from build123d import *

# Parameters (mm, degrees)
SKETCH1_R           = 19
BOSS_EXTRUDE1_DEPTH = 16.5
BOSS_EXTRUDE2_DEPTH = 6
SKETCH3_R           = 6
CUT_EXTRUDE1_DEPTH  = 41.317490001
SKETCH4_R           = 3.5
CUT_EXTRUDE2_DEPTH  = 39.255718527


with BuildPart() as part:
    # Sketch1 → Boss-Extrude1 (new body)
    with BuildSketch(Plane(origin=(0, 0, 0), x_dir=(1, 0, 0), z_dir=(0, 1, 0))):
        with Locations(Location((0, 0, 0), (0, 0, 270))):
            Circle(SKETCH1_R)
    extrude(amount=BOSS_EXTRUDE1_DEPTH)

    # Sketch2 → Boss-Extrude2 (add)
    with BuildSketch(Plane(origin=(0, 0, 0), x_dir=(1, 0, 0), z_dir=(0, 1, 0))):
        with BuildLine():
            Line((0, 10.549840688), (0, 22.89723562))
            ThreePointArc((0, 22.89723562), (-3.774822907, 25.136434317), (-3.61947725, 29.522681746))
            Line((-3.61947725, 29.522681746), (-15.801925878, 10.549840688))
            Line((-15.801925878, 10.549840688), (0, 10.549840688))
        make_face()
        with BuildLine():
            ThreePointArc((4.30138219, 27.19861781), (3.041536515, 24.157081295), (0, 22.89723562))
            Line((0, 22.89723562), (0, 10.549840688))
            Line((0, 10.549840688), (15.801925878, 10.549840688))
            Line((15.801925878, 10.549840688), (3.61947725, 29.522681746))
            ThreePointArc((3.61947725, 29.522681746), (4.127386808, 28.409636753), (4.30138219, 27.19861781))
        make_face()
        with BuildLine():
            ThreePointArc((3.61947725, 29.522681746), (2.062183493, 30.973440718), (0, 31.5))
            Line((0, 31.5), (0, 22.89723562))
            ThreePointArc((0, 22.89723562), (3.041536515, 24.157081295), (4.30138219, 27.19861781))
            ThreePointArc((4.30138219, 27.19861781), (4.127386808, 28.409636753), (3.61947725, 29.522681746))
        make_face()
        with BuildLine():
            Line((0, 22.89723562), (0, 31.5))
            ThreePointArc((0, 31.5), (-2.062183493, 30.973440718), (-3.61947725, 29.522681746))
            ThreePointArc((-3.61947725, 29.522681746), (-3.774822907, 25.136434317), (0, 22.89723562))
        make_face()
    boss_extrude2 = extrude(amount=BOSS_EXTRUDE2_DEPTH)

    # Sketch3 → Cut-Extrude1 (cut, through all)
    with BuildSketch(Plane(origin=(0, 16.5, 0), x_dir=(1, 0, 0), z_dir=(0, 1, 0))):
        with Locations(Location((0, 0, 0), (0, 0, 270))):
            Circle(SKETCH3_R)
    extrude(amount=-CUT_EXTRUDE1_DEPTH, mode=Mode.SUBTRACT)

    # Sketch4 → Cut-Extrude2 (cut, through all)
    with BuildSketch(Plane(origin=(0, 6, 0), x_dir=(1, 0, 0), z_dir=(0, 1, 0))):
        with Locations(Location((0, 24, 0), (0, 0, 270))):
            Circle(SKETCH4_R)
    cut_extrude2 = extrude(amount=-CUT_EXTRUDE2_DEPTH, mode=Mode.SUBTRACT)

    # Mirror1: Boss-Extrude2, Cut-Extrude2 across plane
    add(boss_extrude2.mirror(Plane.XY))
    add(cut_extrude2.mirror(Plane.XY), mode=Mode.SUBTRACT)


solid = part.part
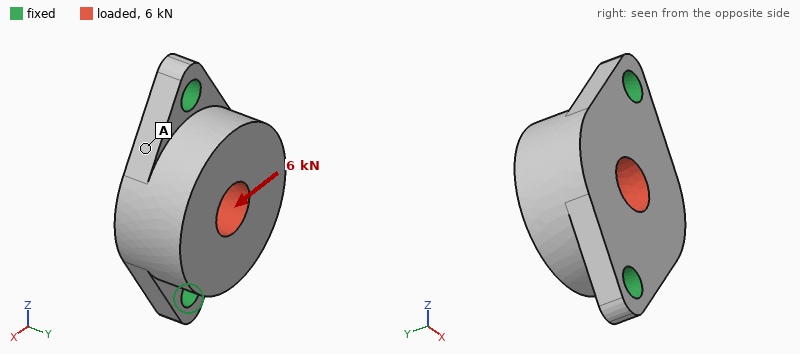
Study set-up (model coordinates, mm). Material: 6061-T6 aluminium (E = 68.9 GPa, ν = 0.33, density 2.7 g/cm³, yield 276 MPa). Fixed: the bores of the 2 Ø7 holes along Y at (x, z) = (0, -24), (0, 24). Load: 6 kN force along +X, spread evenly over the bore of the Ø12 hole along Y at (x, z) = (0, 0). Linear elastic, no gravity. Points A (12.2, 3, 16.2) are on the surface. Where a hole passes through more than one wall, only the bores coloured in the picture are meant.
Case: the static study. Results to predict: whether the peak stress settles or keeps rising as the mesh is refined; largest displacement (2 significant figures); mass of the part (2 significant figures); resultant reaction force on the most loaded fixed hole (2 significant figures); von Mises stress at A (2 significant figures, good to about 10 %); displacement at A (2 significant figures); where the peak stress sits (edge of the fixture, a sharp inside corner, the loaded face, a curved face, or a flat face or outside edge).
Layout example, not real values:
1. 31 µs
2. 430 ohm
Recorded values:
1. keeps rising
2. 68 µm
3. 50 g
4. 3.0 kN
5. 40 MPa
6. 29 µm
7. edge of the fixture
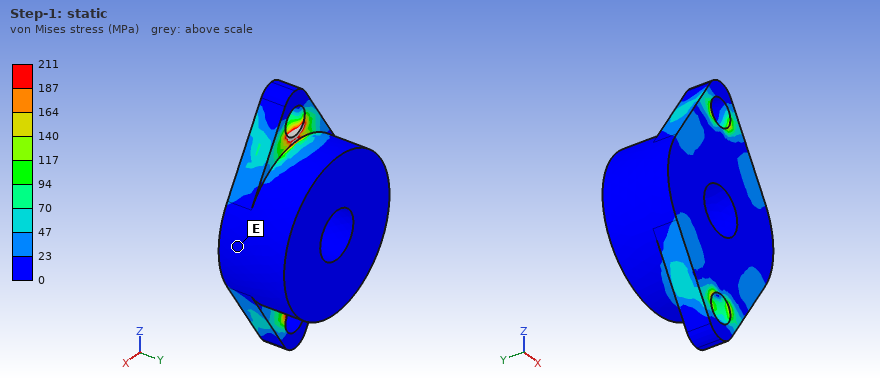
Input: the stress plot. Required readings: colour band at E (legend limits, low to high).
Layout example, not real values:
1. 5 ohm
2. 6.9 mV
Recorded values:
1. 0 to 23 MPa
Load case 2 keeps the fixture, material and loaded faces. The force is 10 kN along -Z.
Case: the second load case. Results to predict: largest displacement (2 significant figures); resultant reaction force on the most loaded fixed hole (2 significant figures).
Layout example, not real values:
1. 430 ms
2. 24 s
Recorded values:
1. 13 µm
2. 5.2 kN
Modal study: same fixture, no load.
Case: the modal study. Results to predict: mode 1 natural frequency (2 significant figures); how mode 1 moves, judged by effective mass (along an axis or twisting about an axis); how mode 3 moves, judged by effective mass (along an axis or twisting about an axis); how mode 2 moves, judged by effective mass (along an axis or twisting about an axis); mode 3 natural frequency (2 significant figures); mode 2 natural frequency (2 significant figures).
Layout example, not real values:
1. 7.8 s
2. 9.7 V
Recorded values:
1. 6600 Hz
2. along X
3. along X
4. along Y
5. 20 kHz
6. 13 kHz
